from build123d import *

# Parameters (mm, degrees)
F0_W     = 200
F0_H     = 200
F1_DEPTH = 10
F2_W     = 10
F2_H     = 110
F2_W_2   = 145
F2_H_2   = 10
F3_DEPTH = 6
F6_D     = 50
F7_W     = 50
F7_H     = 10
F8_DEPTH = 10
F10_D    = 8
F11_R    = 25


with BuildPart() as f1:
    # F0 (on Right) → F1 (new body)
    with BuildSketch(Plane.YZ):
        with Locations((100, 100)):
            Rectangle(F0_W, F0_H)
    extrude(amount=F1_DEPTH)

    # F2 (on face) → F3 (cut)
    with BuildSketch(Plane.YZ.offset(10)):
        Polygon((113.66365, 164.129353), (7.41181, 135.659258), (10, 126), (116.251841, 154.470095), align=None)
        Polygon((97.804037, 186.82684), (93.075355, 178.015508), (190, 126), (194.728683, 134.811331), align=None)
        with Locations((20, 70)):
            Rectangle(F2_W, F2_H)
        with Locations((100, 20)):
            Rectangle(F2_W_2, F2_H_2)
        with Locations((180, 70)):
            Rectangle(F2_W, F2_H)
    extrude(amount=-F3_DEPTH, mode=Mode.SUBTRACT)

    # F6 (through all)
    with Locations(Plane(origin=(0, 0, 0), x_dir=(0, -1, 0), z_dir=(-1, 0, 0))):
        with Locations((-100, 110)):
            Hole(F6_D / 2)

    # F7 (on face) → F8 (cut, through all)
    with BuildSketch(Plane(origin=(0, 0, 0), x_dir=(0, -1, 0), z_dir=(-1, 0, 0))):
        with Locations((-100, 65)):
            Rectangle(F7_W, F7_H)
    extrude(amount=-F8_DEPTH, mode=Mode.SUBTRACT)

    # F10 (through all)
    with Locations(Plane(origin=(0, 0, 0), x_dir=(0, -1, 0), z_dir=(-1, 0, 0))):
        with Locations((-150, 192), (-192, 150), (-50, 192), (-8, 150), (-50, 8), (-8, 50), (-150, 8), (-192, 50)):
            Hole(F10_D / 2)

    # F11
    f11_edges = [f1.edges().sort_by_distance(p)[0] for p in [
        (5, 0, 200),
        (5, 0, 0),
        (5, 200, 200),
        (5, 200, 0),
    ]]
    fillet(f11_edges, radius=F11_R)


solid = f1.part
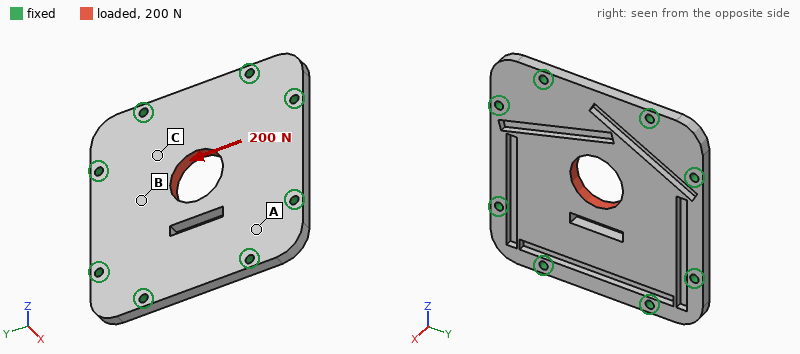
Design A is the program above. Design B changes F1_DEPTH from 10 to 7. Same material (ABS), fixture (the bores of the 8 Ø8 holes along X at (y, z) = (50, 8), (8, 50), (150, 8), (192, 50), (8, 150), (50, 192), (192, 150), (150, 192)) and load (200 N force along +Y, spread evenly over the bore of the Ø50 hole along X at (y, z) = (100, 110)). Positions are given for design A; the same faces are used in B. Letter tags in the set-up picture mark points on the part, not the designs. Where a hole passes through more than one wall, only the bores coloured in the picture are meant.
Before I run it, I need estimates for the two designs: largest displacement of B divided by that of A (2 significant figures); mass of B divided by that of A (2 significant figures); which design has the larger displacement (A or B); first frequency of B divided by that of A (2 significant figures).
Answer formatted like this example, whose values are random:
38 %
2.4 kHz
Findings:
1.2
0.72
B
0.76
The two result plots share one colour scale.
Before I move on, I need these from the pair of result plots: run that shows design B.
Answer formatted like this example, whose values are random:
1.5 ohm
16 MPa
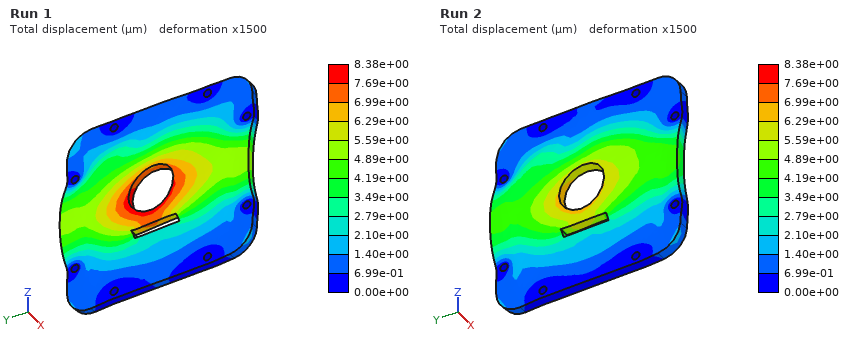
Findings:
Run 1
